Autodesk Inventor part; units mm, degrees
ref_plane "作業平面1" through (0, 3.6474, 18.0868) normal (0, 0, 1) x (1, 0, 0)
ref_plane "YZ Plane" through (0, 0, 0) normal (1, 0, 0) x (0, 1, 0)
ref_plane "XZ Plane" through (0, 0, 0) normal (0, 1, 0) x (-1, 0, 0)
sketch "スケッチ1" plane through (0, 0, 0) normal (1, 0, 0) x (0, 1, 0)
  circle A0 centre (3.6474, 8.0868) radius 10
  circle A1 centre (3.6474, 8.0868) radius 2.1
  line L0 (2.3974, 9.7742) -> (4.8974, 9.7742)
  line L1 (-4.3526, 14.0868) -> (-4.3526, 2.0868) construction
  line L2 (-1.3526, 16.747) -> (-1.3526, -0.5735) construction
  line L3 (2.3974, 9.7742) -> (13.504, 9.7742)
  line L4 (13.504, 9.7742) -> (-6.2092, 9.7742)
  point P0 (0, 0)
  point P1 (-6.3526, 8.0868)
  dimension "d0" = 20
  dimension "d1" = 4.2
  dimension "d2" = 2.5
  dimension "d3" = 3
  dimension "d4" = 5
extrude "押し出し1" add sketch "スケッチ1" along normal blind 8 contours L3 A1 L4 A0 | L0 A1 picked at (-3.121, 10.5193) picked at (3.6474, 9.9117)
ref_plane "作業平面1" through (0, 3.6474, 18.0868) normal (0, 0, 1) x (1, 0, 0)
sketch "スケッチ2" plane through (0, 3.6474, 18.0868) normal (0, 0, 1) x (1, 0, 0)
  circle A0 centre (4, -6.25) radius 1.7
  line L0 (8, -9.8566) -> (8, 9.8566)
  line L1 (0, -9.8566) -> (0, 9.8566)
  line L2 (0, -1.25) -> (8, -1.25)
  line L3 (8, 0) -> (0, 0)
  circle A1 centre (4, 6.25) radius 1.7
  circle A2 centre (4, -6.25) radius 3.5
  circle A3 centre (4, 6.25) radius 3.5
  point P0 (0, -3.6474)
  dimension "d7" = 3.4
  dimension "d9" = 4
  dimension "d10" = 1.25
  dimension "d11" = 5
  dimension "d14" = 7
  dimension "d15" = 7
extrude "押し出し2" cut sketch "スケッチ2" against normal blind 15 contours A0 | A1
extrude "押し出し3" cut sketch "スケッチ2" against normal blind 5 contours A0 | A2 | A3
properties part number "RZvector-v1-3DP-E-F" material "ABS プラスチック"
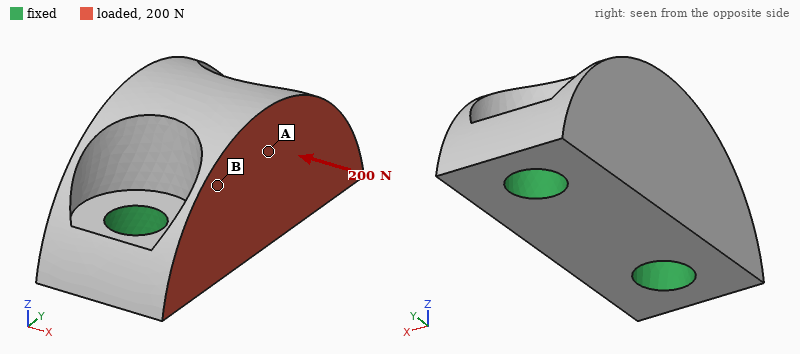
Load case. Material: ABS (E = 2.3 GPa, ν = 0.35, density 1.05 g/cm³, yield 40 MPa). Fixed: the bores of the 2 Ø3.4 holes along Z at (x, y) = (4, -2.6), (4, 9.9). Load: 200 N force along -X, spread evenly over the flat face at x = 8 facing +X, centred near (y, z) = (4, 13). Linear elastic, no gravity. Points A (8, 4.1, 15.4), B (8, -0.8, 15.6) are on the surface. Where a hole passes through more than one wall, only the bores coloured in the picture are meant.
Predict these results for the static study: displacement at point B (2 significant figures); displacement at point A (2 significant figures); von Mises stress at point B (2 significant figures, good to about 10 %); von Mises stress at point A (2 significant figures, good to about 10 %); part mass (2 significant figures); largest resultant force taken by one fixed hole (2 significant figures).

55 µm
42 µm
8.9 MPa
3.1 MPa
0.77 g
100 N
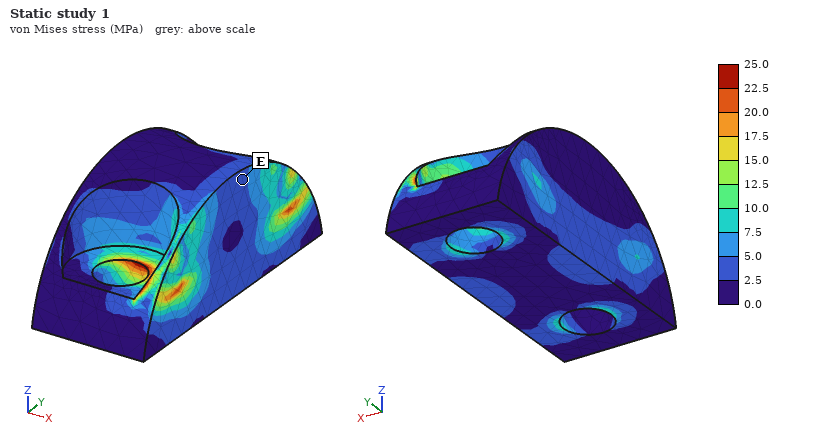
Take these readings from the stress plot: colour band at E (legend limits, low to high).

2.5 to 5.0 MPa
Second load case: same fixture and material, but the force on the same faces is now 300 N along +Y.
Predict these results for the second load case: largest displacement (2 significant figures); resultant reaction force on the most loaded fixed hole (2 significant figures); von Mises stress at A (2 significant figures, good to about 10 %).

66 µm
170 N
9.3 MPa
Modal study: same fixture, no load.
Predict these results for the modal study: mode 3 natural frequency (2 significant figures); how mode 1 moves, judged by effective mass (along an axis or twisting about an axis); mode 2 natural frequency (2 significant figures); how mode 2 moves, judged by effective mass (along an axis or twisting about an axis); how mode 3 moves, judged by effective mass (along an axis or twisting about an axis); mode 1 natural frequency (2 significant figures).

25 kHz
along X
23 kHz
along Z
along Y
13 kHz
